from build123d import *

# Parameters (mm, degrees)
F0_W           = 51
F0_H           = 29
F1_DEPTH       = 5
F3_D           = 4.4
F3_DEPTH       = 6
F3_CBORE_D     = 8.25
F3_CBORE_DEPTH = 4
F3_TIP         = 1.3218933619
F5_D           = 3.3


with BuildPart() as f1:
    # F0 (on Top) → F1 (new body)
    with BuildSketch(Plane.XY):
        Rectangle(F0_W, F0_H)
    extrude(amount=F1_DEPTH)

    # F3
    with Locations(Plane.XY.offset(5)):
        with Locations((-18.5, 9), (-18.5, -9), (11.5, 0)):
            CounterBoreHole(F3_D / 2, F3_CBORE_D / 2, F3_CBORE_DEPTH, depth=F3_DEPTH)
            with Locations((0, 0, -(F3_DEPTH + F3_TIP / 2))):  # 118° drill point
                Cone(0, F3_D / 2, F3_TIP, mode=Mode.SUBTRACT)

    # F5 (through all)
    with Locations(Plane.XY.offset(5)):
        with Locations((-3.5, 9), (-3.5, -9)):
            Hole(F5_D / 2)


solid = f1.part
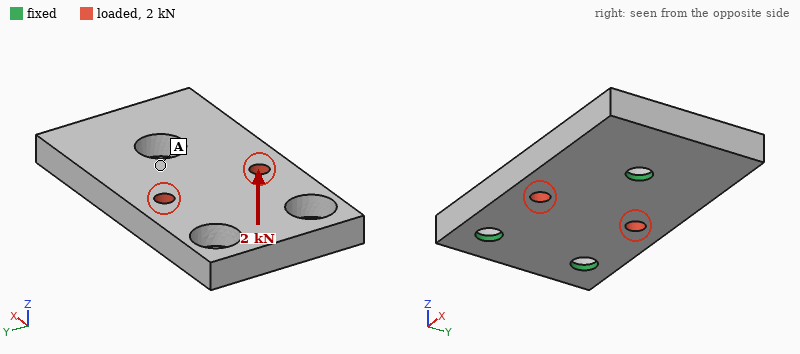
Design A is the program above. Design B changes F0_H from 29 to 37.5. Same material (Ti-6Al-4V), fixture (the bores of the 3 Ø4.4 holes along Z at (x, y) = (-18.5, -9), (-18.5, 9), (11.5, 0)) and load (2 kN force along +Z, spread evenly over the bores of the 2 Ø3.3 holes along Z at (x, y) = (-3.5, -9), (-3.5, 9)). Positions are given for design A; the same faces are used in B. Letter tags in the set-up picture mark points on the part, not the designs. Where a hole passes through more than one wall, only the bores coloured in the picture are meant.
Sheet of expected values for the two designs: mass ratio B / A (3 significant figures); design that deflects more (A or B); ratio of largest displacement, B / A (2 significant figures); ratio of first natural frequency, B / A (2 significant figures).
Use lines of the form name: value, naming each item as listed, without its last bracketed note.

mass ratio B / A: 1.33
design that deflects more: A
ratio of largest displacement, B / A: 0.86
ratio of first natural frequency, B / A: 0.75
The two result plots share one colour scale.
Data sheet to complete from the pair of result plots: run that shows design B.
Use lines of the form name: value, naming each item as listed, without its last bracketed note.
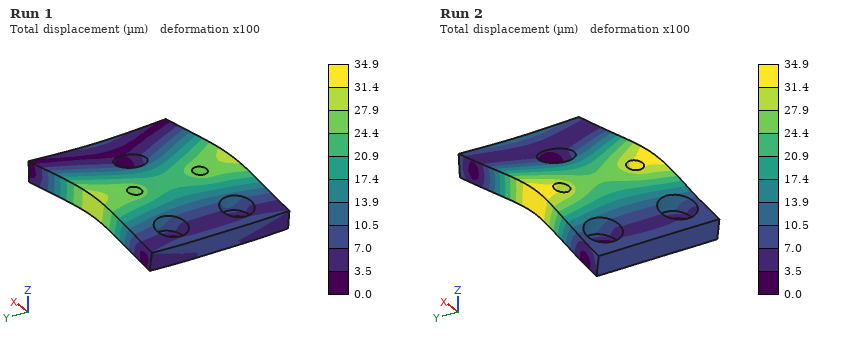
run that shows design B: Run 1
